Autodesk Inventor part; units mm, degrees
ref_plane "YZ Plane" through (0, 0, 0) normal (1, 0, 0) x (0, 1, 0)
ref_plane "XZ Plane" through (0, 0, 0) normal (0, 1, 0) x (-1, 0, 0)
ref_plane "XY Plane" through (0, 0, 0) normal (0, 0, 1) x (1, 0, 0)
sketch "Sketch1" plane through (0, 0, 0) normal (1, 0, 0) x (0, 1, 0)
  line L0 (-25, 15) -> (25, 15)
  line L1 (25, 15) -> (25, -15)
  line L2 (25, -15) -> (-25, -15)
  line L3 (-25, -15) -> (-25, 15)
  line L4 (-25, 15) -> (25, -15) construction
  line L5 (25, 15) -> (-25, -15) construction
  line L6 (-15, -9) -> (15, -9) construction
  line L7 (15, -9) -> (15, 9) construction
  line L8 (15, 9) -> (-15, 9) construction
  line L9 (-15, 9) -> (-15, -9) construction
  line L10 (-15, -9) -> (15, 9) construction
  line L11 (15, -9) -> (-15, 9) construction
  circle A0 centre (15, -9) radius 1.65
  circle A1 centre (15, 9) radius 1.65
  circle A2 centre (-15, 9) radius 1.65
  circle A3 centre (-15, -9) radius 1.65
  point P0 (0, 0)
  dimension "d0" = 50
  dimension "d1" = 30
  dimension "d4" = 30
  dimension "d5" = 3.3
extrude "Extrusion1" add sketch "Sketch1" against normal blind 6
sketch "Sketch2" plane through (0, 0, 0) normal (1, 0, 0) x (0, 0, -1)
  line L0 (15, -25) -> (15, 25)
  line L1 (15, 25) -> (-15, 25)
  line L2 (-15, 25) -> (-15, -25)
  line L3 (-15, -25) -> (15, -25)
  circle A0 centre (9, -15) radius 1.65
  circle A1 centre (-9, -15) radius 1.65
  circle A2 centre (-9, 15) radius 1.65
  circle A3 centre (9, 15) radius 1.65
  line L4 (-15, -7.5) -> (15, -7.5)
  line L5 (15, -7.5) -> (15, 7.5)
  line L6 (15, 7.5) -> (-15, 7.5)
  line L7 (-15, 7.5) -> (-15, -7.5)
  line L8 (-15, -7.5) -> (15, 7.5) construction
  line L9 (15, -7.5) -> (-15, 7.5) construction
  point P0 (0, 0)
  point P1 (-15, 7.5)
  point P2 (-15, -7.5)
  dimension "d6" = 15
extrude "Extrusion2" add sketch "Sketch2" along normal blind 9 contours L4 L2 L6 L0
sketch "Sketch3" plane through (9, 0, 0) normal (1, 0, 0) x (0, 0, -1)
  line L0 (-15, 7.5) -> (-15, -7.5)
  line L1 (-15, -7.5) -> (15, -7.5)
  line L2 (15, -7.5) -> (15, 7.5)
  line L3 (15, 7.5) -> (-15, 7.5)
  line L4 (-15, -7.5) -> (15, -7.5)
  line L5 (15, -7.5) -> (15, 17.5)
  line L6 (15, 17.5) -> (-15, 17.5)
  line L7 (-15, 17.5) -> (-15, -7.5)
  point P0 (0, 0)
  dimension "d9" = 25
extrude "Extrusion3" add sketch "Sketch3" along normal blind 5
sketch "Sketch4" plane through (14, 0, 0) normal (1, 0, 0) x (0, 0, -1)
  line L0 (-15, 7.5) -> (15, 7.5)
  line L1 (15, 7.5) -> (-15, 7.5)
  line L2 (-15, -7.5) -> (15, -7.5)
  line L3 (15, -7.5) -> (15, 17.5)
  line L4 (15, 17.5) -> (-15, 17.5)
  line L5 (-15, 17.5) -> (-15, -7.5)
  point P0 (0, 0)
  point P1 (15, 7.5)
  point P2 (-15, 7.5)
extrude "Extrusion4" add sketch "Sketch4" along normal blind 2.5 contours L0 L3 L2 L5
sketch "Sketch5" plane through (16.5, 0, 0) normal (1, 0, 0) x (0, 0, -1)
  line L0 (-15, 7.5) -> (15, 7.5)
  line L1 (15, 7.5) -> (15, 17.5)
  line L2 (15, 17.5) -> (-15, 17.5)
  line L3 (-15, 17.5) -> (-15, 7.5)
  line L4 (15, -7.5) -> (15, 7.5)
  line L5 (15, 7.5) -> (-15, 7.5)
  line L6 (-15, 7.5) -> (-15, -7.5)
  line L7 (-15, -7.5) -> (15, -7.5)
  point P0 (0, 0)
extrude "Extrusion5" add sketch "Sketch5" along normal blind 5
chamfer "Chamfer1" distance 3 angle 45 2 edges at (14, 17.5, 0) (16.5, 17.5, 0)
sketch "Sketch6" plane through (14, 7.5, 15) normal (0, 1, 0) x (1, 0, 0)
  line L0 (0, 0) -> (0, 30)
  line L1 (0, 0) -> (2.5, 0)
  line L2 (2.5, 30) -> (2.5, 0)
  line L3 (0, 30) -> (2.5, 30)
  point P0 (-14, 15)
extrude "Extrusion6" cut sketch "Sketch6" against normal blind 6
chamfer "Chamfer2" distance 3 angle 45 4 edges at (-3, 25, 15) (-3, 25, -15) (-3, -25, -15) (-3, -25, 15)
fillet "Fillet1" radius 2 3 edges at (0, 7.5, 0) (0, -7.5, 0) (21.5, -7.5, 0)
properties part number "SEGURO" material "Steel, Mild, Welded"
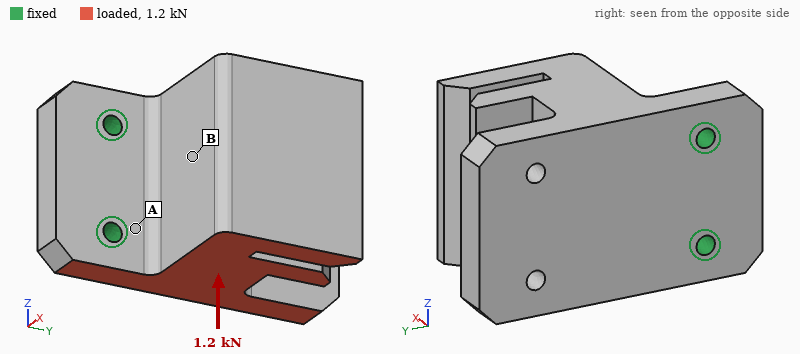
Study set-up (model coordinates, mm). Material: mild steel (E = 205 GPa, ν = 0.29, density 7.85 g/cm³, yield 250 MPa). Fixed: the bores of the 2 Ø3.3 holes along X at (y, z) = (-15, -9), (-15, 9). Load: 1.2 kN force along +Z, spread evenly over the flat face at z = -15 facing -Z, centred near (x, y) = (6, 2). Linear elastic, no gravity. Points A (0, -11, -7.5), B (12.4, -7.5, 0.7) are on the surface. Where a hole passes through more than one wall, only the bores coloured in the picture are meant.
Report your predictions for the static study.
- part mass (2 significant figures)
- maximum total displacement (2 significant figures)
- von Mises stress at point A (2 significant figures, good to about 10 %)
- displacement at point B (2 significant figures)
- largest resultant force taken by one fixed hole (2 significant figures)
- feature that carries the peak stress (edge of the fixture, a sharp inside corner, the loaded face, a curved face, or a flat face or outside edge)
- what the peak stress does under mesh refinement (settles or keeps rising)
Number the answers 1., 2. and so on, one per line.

1. 160 g
2. 8.1 µm
3. 32 MPa
4. 3.9 µm
5. 1.3 kN
6. edge of the fixture
7. keeps rising
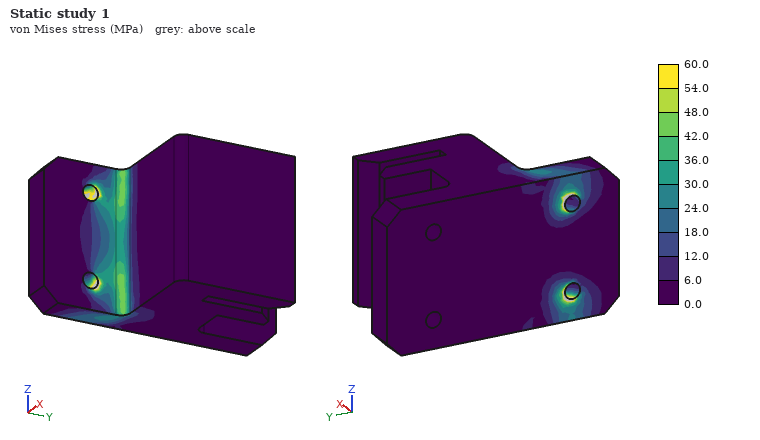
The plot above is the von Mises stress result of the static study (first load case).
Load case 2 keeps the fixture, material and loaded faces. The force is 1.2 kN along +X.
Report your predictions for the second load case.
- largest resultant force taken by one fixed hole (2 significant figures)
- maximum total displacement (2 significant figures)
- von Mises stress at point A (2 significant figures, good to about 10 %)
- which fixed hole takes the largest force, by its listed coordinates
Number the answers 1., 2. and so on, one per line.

1. 1.4 kN
2. 63 µm
3. 110 MPa
4. (-15, -9)
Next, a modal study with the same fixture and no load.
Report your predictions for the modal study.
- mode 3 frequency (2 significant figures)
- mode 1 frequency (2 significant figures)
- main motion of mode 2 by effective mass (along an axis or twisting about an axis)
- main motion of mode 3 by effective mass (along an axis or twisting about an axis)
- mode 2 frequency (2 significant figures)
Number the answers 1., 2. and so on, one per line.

1. 8900 Hz
2. 2000 Hz
3. along Z
4. along Z
5. 5900 Hz
